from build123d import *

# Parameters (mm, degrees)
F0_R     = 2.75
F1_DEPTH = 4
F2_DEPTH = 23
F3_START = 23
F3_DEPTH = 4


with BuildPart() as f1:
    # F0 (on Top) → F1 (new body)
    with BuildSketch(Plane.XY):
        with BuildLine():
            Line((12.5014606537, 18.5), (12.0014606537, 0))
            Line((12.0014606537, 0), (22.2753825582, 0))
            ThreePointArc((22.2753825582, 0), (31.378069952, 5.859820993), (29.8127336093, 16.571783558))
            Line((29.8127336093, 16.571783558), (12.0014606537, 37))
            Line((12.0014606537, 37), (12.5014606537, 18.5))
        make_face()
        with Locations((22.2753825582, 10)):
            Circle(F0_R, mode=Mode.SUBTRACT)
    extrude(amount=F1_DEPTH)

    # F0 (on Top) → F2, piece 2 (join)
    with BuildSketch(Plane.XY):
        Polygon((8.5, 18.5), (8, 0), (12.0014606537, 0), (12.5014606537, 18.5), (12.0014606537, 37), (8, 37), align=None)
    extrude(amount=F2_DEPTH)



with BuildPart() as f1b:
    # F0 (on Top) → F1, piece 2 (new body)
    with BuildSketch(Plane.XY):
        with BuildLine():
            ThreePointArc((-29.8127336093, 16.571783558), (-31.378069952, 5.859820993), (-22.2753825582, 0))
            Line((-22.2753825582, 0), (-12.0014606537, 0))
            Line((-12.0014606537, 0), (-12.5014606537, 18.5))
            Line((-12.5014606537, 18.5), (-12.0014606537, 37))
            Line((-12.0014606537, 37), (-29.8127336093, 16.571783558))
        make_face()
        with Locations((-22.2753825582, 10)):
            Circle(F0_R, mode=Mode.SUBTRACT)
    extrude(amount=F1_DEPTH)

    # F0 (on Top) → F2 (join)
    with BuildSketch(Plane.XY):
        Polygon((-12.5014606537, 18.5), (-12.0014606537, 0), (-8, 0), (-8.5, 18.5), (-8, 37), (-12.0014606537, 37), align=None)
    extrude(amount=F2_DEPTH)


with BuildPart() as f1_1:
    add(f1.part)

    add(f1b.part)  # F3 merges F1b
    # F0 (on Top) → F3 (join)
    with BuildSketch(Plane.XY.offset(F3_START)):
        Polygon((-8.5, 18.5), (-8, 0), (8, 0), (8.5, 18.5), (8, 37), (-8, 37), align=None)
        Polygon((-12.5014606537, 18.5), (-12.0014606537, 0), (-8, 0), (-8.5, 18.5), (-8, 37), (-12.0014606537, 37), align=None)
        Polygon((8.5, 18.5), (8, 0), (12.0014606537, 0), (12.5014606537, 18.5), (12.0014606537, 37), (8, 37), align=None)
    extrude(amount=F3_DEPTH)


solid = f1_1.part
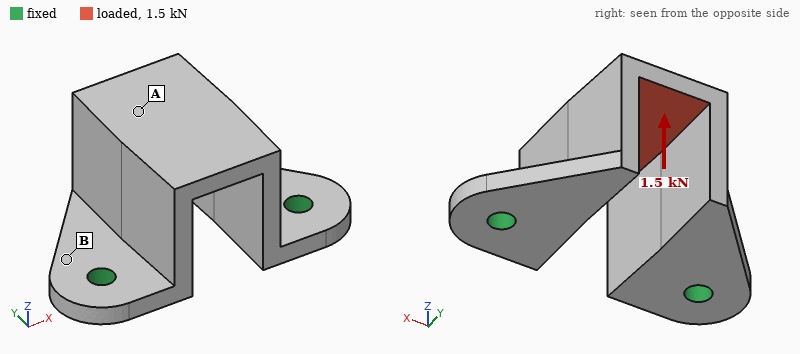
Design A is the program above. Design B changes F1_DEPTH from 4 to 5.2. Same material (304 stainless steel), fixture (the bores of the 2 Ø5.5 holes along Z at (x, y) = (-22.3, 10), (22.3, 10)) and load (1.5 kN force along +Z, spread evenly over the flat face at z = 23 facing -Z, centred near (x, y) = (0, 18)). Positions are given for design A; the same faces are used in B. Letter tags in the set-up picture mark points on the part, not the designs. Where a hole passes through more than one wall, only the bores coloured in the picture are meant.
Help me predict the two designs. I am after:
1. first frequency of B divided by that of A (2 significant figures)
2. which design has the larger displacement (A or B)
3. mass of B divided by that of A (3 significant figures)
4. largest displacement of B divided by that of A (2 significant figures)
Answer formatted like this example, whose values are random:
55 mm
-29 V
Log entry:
1.4
A
1.08
0.57
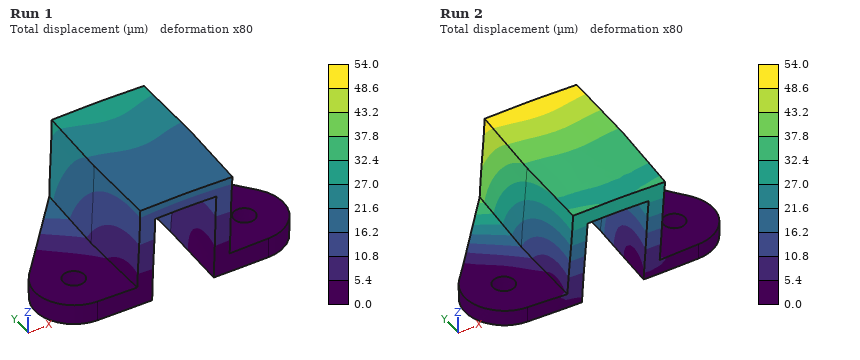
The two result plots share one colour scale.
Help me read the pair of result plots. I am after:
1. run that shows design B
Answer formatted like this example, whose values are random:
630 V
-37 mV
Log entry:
Run 1
